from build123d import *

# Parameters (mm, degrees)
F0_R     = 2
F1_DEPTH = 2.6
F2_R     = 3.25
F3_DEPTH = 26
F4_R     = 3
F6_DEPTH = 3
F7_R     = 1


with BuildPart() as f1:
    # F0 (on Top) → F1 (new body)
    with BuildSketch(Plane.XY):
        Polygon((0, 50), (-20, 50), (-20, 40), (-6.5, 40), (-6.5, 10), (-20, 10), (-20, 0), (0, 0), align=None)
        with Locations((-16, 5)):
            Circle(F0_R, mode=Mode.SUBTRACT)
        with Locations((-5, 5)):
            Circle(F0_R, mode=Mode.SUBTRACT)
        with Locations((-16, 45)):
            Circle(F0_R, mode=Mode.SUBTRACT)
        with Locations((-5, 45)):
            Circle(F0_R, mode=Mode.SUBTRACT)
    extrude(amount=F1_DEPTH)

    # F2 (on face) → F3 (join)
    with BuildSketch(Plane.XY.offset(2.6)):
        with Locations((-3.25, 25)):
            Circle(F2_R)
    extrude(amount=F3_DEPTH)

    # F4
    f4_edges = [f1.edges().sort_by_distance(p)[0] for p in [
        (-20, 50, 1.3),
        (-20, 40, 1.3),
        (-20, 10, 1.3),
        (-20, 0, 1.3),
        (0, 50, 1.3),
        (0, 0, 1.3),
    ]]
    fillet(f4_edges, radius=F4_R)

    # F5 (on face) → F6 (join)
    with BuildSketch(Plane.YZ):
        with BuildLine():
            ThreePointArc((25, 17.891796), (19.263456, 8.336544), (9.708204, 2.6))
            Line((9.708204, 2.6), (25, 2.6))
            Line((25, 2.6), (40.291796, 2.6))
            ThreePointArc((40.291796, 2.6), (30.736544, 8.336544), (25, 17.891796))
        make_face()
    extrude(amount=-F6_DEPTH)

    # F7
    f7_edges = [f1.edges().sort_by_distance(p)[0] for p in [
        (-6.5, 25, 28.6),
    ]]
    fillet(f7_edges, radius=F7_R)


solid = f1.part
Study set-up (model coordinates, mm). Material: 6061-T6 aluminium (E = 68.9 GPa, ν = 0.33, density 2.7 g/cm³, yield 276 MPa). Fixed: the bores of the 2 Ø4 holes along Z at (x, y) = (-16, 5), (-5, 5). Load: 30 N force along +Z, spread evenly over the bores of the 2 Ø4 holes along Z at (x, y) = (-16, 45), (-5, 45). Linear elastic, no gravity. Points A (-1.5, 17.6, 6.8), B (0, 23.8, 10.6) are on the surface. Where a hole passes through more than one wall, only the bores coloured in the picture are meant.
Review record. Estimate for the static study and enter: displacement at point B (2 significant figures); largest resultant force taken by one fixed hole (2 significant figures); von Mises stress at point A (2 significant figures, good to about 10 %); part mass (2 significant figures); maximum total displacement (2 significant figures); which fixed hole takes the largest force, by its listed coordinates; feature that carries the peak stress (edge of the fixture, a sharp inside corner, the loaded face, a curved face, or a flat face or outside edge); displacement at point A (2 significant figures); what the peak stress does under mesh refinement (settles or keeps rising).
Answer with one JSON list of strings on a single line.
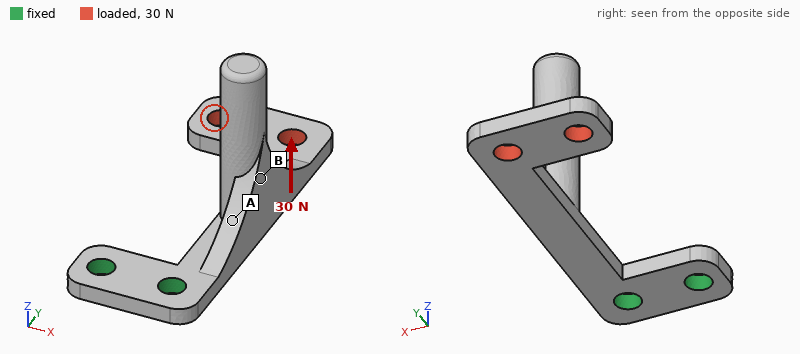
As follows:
["0.17 mm", "40 N", "28 MPa", "6.8 g", "0.55 mm", "(-5, 5)", "edge of the fixture", "0.094 mm", "keeps rising"]
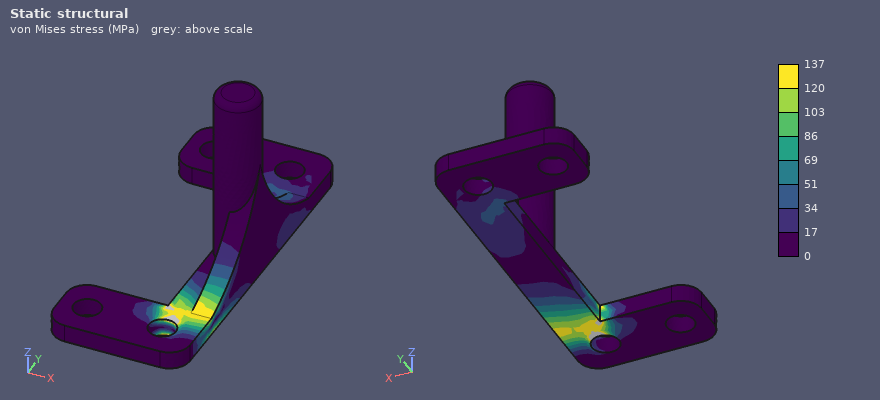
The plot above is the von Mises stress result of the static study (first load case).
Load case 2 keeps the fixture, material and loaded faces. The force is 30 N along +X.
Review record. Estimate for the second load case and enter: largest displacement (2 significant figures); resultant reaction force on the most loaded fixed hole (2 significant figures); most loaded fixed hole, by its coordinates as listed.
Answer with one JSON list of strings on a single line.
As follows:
["0.16 mm", "62 N", "(-16, 5)"]
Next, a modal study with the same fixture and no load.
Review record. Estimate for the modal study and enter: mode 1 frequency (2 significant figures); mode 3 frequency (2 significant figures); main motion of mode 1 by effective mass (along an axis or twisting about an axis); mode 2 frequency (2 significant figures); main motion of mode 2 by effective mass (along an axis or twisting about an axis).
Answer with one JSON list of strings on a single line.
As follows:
["860 Hz", "2100 Hz", "along Z", "1500 Hz", "along X"]
